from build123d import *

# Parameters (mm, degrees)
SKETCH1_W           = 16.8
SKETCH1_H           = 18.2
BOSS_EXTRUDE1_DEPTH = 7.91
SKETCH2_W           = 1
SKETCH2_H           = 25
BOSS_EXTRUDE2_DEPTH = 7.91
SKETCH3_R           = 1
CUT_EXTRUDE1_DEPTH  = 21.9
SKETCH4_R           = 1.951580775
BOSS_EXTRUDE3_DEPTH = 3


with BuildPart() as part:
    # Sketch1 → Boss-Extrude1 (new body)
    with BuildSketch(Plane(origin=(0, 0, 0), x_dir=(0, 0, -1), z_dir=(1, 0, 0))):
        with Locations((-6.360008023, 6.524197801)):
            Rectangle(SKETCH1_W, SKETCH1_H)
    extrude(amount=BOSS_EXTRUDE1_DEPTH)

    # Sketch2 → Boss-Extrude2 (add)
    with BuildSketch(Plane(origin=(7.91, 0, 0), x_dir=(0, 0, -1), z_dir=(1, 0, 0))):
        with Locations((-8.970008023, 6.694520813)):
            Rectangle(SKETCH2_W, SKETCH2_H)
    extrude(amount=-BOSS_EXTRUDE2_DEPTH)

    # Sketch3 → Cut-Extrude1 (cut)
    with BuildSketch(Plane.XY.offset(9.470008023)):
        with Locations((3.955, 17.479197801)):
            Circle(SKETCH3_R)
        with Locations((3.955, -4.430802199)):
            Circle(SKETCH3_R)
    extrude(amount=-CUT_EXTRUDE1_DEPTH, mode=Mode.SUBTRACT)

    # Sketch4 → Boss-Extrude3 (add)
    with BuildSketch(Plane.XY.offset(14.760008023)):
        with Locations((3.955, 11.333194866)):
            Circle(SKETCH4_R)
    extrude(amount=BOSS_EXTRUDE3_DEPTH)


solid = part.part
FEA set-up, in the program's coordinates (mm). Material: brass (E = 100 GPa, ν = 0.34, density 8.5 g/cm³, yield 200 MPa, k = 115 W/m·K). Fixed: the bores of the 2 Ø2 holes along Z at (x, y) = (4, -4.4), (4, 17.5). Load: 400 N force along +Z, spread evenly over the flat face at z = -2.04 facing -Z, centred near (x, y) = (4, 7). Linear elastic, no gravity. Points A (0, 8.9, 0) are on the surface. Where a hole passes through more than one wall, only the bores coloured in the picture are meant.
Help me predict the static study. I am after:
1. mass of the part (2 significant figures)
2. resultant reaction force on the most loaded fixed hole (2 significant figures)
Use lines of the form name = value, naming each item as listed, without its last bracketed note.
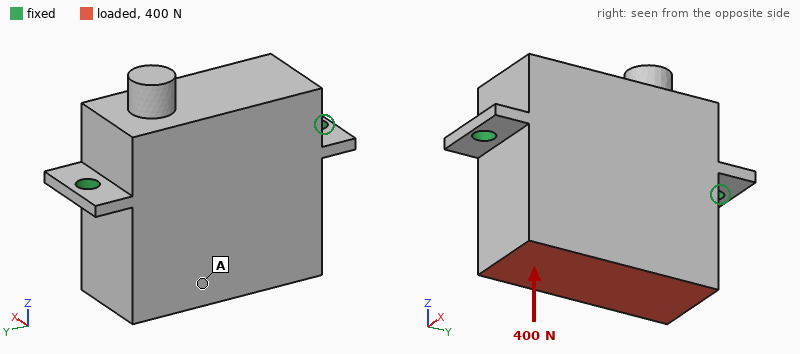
mass of the part = 21 g
resultant reaction force on the most loaded fixed hole = 200 N
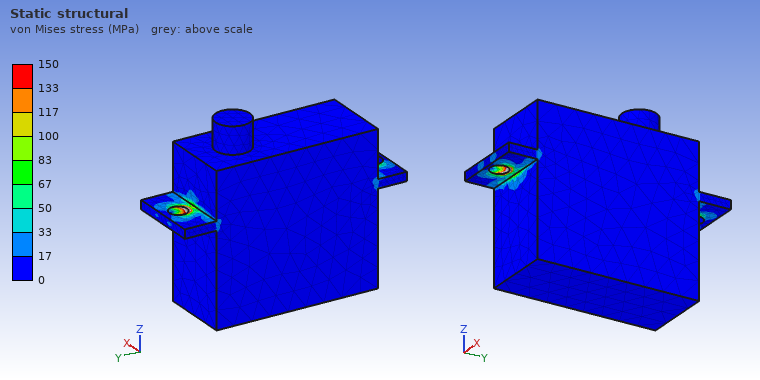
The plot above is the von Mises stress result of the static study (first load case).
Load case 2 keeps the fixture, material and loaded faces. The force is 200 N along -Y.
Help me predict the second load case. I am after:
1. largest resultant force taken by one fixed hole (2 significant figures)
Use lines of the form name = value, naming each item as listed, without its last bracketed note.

largest resultant force taken by one fixed hole = 150 N
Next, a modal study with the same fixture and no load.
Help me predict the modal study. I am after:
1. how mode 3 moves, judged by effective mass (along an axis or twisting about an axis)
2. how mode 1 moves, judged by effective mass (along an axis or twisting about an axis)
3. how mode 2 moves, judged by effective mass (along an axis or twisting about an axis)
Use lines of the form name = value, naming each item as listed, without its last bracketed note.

how mode 3 moves, judged by effective mass = along Y
how mode 1 moves, judged by effective mass = along X
how mode 2 moves, judged by effective mass = along Z
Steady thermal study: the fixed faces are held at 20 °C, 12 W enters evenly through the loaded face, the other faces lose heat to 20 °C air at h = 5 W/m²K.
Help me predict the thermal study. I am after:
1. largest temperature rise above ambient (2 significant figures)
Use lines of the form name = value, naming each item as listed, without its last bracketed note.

largest temperature rise above ambient = 26 K
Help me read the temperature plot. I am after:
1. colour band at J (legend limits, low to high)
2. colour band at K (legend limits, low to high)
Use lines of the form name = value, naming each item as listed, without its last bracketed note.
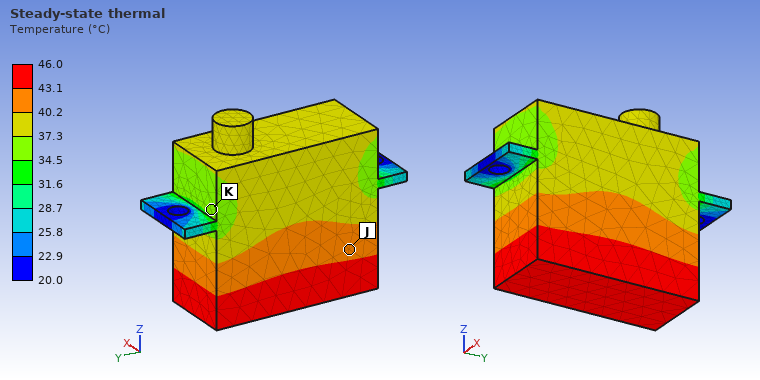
colour band at J = 40.2 to 43.1 °C
colour band at K = 34.5 to 37.3 °C
